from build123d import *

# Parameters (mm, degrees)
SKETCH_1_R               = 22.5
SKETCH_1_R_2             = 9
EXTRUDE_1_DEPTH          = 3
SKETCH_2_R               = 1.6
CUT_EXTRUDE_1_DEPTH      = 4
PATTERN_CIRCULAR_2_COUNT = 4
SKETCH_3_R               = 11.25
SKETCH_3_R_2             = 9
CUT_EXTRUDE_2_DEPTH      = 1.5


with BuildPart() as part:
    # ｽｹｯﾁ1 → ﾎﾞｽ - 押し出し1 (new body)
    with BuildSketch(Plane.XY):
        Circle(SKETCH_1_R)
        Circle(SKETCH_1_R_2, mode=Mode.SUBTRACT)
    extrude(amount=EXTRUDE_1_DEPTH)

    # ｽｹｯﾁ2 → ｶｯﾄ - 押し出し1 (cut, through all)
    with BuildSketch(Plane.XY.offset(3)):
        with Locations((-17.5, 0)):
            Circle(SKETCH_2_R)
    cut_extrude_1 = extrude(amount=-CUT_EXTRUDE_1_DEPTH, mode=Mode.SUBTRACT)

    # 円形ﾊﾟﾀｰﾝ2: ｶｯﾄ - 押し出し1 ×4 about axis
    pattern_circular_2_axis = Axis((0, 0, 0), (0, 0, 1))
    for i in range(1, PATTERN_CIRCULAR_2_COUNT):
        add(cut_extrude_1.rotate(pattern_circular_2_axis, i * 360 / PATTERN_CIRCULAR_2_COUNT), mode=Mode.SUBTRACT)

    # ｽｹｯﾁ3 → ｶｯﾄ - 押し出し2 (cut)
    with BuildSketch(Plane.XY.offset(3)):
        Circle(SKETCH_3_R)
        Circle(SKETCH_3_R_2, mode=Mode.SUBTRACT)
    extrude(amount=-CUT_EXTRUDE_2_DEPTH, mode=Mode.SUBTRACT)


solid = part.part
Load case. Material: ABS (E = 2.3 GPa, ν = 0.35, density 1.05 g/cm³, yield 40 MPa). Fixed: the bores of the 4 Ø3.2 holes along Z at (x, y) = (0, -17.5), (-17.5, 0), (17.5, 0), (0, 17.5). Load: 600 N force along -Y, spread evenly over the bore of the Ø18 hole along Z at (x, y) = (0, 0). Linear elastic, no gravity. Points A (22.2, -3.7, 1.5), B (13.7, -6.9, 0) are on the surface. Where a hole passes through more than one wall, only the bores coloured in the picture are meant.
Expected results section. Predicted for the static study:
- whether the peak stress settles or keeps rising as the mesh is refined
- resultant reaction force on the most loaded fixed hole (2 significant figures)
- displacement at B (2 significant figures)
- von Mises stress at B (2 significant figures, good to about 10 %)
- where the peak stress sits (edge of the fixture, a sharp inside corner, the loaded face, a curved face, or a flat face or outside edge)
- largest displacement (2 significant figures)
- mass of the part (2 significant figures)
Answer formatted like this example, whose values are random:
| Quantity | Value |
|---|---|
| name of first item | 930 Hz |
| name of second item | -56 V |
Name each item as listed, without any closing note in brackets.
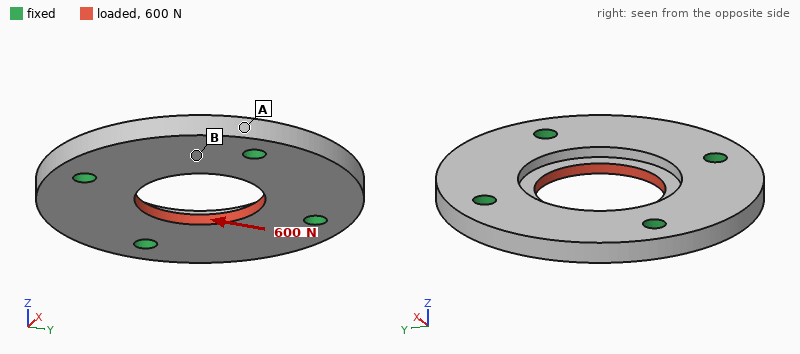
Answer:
| Quantity | Value |
|---|---|
| whether the peak stress settles or keeps rising as the mesh is refined | keeps rising |
| resultant reaction force on the most loaded fixed hole | 160 N |
| displacement at B | 22 µm |
| von Mises stress at B | 3.3 MPa |
| where the peak stress sits | edge of the fixture |
| largest displacement | 53 µm |
| mass of the part | 3.9 g |
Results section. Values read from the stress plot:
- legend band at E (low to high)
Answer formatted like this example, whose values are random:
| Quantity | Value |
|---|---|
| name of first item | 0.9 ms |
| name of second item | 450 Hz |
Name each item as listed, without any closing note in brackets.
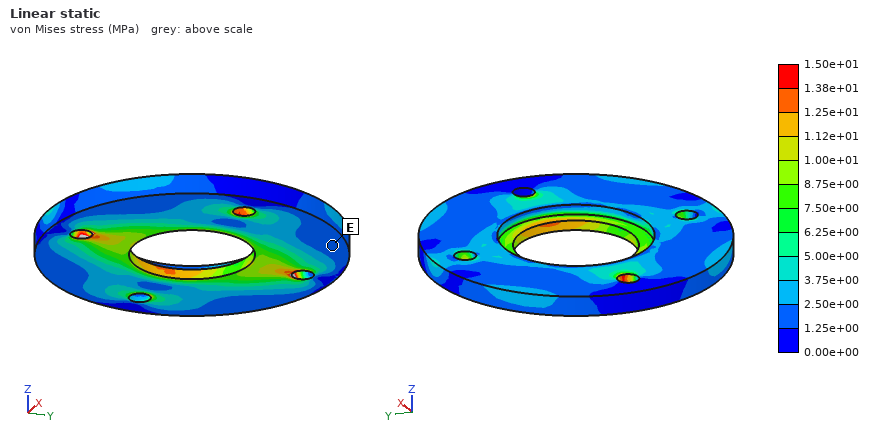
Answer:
| Quantity | Value |
|---|---|
| legend band at E | 1.25e+00 to 2.50e+00 MPa |
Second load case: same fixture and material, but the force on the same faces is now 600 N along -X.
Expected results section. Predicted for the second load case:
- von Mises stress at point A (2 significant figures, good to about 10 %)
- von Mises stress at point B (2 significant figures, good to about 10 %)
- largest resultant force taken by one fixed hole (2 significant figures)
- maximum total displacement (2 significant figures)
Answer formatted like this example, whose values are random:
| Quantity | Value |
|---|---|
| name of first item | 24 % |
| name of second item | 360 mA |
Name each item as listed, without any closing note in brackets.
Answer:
| Quantity | Value |
|---|---|
| von Mises stress at point A | 1.4 MPa |
| von Mises stress at point B | 4.5 MPa |
| largest resultant force taken by one fixed hole | 160 N |
| maximum total displacement | 53 µm |
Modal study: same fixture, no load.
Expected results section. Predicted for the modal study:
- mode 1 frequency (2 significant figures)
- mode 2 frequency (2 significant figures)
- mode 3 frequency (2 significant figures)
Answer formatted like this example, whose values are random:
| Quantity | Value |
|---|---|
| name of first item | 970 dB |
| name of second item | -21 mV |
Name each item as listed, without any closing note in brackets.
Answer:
| Quantity | Value |
|---|---|
| mode 1 frequency | 5100 Hz |
| mode 2 frequency | 5400 Hz |
| mode 3 frequency | 5400 Hz |
